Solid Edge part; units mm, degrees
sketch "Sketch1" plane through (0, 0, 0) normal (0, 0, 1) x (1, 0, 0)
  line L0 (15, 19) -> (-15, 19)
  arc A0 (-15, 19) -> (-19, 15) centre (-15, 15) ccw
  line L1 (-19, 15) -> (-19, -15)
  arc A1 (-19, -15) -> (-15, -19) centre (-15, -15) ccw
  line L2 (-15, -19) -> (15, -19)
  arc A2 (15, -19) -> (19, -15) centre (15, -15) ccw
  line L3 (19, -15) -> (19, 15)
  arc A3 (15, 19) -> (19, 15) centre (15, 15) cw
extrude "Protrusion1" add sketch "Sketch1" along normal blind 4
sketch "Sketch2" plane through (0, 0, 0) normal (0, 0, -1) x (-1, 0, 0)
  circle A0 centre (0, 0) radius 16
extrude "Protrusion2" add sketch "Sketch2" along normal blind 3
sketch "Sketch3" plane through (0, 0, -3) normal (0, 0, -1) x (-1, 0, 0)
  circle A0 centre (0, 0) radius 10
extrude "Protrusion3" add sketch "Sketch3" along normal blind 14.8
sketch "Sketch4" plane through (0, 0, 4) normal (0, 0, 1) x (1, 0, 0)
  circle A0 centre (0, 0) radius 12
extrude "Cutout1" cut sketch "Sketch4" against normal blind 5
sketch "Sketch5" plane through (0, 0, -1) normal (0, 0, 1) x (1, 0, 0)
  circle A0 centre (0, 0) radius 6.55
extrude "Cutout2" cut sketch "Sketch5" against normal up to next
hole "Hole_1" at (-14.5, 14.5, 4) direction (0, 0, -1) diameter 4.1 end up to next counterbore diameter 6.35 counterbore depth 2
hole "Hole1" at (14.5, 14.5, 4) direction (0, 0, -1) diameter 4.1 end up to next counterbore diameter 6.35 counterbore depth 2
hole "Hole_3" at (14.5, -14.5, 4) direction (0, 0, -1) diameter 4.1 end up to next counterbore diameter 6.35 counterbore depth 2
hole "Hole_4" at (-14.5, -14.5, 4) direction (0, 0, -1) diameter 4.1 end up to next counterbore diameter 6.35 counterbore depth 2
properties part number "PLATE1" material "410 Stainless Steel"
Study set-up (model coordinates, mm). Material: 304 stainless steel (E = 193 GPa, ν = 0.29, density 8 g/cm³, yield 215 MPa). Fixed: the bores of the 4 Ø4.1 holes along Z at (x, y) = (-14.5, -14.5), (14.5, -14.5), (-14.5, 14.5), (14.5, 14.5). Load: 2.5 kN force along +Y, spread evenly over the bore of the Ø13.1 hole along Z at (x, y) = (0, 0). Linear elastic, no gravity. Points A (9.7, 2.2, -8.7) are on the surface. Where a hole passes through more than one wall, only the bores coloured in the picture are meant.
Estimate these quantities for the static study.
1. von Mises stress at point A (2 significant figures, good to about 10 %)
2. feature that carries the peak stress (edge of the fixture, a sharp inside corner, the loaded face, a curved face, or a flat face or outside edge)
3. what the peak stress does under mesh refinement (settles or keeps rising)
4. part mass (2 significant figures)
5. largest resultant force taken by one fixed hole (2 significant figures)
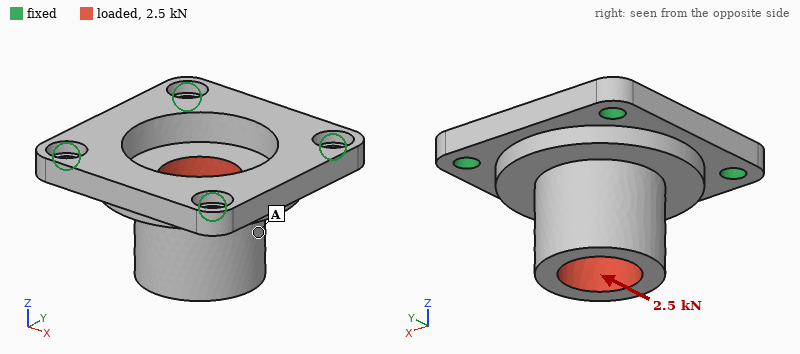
14 MPa
edge of the fixture
keeps rising
63 g
820 N
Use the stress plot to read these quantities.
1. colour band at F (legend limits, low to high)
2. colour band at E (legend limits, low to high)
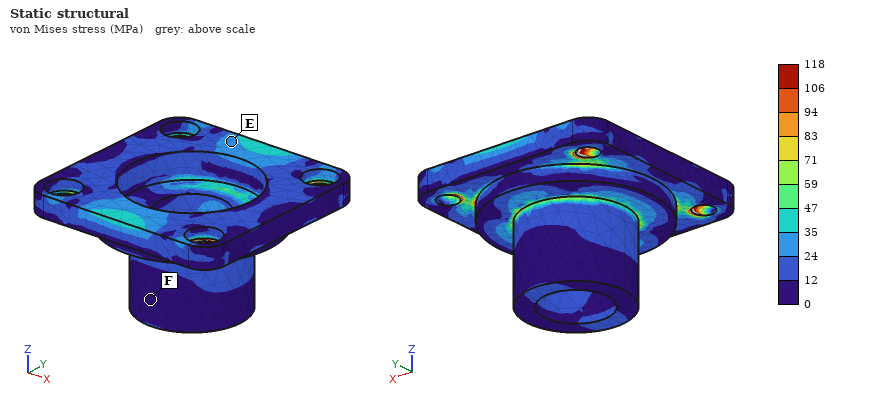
0 to 12 MPa
24 to 35 MPa
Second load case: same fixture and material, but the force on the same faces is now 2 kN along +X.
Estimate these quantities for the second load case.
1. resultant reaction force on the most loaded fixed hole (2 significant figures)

660 N
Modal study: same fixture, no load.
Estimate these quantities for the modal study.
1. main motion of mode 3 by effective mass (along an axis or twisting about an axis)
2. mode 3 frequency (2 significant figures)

along Z
14 kHz
